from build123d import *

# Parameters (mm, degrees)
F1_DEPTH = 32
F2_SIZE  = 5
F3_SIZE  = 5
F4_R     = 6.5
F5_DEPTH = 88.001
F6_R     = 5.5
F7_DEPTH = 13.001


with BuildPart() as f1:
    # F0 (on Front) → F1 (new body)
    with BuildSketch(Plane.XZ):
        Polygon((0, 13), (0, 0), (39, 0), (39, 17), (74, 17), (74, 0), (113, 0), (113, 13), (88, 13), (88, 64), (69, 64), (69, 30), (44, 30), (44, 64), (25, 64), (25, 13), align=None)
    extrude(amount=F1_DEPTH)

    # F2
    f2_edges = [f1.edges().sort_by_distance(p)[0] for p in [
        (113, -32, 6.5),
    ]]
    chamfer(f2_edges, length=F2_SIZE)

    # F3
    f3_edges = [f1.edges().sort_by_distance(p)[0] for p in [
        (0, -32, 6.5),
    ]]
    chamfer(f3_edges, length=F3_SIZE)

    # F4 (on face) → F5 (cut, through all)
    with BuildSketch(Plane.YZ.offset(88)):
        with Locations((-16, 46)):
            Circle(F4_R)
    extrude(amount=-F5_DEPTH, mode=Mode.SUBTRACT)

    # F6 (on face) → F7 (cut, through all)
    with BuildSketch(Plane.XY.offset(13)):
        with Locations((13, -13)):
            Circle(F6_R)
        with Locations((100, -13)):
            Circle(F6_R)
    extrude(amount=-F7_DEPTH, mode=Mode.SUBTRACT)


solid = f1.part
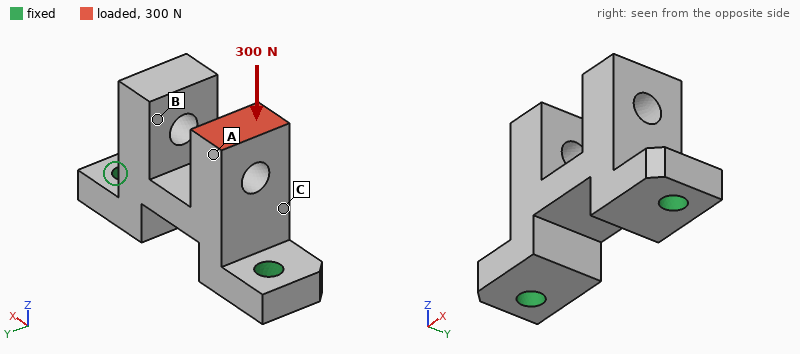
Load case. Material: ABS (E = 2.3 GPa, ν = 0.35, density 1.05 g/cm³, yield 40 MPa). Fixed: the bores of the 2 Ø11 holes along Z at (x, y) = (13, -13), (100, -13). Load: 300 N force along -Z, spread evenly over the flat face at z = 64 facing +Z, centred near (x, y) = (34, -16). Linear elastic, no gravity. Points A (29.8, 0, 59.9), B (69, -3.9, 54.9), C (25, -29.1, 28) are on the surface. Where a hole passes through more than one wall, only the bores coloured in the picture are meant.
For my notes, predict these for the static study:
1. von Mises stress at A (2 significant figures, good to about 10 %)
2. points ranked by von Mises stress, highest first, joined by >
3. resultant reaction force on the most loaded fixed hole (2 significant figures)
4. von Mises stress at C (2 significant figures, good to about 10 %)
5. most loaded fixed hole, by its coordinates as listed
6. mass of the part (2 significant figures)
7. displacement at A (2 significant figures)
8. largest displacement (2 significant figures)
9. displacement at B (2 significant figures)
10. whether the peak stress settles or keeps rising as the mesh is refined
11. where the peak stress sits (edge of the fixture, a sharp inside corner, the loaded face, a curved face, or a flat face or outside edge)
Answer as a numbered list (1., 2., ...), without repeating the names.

1. 0.50 MPa
2. C > A > B
3. 270 N
4. 0.78 MPa
5. (13, -13)
6. 100 g
7. 34 µm
8. 45 µm
9. 14 µm
10. keeps rising
11. edge of the fixture
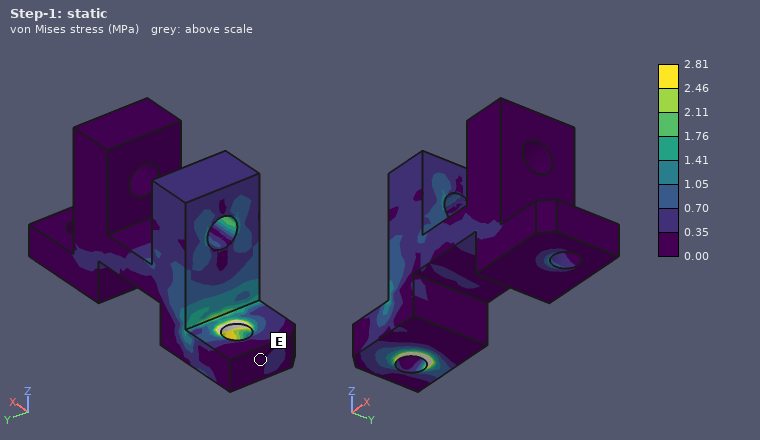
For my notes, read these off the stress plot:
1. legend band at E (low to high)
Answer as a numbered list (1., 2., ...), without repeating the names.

1. 0.00 to 0.35 MPa
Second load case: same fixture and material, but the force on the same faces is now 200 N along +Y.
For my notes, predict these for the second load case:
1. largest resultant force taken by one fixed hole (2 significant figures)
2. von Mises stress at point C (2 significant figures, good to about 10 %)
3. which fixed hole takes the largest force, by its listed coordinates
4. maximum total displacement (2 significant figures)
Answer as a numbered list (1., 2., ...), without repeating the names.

1. 140 N
2. 2.2 MPa
3. (13, -13)
4. 0.51 mm
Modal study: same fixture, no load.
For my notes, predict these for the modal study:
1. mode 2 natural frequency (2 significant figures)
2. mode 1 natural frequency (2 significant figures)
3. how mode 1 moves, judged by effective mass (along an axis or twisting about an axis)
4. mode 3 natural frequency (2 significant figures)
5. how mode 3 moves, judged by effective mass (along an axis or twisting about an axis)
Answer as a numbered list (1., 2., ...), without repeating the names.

1. 1300 Hz
2. 790 Hz
3. along Y
4. 1600 Hz
5. along X
